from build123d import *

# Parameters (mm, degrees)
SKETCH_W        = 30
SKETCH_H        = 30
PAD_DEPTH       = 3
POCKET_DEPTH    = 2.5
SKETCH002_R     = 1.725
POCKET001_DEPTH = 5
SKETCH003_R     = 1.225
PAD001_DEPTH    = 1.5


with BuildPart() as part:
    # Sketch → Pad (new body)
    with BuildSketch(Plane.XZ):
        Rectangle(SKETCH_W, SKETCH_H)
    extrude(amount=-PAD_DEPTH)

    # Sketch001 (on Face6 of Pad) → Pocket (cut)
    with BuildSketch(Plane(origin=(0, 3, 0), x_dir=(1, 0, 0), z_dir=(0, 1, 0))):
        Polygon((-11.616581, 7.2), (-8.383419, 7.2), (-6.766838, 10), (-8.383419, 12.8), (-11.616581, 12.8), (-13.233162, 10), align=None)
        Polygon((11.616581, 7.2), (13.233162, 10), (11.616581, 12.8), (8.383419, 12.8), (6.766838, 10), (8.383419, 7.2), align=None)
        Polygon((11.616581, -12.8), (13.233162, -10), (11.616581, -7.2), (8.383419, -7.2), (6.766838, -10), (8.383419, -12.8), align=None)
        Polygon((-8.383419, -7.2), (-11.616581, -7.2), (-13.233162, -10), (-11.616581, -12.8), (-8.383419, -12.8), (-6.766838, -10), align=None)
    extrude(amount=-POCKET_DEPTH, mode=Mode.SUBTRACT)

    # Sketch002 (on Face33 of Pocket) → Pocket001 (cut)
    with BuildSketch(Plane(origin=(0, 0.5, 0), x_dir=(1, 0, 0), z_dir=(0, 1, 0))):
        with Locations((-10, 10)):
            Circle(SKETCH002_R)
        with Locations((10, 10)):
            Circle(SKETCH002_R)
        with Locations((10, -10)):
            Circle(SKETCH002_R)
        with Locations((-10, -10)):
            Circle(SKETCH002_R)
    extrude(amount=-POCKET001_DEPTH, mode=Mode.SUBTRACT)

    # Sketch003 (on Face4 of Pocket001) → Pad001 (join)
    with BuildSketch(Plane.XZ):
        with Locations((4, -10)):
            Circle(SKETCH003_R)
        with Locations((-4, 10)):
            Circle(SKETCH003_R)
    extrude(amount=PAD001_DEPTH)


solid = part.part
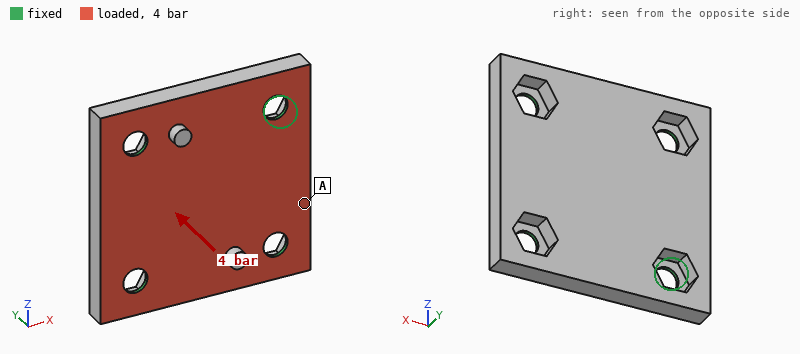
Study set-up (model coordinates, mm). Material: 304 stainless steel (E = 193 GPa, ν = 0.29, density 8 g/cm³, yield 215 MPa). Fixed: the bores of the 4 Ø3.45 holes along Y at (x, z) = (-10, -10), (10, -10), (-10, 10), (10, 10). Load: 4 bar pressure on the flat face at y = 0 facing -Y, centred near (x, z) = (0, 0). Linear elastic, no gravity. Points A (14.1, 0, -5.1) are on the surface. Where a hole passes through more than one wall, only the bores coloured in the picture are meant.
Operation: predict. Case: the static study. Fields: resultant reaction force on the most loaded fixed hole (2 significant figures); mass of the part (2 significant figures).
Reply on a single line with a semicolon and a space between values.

100 N; 19 g
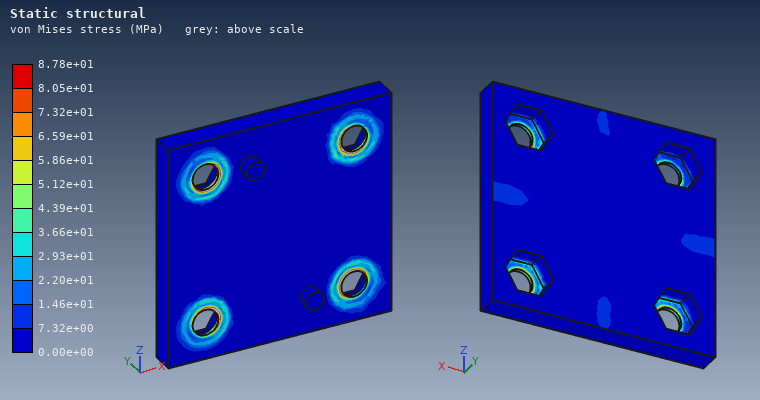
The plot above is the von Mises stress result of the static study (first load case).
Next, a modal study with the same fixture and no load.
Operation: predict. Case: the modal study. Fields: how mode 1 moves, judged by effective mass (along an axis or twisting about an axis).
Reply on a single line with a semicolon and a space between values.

along Y
